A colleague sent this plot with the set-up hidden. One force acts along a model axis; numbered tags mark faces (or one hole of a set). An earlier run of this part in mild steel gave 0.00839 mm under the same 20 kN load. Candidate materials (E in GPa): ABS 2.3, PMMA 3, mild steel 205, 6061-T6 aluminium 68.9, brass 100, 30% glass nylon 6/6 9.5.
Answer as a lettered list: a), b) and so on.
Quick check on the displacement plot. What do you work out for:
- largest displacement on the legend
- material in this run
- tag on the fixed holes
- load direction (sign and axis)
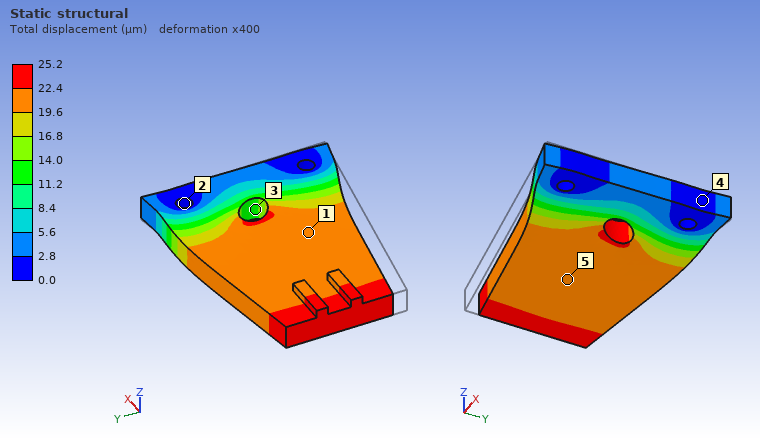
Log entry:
a) 25.2 µm
b) 6061-T6 aluminium
c) 2
d) +Y
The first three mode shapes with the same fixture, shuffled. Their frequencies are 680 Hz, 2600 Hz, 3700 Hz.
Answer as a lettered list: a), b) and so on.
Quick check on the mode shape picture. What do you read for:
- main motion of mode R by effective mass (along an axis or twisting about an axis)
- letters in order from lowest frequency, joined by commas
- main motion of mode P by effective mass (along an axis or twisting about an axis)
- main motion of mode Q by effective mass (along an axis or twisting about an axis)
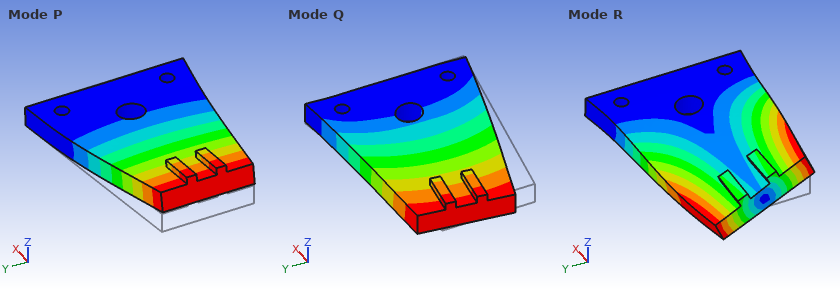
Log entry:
a) twisting about X
b) P, R, Q
c) along Z
d) along Y
